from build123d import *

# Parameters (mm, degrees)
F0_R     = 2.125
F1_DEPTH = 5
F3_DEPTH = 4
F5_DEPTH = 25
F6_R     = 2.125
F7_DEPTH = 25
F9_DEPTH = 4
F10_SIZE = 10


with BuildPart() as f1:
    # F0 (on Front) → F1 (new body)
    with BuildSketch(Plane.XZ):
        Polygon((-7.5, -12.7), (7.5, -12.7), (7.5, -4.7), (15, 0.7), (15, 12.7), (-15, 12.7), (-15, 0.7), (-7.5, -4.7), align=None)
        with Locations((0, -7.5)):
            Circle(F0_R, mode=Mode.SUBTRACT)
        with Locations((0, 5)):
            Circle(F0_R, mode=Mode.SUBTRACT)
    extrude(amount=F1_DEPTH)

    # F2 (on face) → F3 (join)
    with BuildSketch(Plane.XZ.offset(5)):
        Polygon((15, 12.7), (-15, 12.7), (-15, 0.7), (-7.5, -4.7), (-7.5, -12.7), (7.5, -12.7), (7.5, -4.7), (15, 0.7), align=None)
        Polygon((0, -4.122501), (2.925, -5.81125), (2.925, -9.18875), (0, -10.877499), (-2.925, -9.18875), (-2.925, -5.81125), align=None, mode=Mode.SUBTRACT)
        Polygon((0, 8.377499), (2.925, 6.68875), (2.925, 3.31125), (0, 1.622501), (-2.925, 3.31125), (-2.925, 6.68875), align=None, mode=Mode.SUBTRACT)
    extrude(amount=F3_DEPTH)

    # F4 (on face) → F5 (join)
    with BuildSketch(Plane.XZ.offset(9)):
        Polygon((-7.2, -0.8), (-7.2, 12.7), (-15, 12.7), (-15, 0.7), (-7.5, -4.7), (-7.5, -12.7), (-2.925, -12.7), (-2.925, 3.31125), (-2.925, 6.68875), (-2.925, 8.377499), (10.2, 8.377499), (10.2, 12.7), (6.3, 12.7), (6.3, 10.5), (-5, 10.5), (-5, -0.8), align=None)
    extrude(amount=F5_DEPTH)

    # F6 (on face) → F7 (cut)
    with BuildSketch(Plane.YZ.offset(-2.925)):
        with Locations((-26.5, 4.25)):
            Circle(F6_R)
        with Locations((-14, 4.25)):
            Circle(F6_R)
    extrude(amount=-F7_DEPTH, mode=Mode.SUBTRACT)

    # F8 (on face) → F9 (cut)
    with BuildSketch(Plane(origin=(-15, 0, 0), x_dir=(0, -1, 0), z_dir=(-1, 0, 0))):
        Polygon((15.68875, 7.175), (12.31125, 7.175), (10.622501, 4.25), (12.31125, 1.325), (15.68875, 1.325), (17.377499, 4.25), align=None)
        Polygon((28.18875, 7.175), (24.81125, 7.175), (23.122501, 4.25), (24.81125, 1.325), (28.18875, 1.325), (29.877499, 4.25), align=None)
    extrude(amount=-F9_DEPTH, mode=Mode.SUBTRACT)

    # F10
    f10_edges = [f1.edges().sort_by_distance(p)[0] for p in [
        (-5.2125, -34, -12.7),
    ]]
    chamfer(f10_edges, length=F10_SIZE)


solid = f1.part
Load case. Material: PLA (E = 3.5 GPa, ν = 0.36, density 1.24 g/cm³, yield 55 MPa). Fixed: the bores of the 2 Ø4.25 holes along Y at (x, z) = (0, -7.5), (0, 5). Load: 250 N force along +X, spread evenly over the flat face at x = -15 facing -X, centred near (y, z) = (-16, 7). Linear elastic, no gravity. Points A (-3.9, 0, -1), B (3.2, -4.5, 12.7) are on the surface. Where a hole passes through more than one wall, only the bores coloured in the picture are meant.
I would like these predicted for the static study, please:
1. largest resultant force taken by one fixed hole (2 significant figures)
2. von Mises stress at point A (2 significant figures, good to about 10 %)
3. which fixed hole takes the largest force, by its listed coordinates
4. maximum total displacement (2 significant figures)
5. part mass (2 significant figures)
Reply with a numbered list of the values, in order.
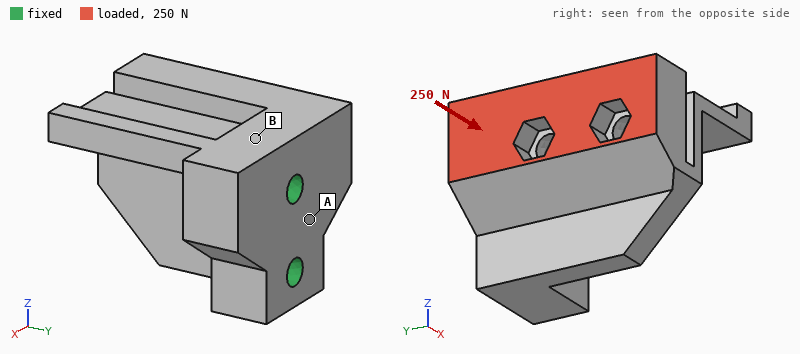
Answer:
1. 260 N
2. 8.0 MPa
3. (0, 5)
4. 0.55 mm
5. 13 g
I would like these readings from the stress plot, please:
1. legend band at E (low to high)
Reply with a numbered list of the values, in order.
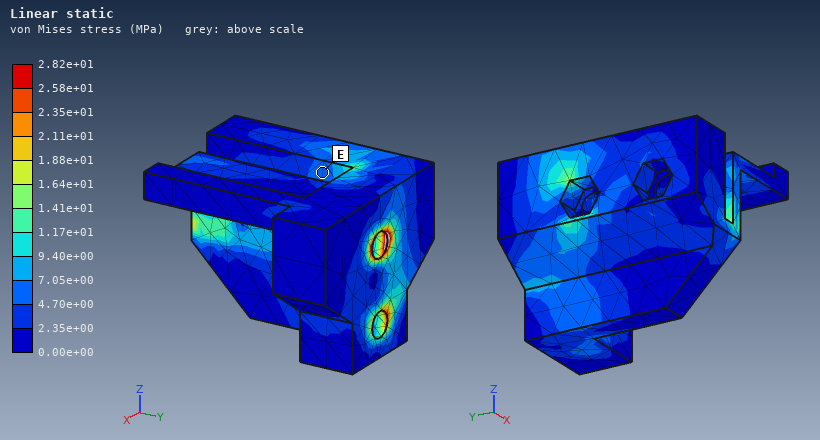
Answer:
1. 4.70e+00 to 7.05e+00 MPa
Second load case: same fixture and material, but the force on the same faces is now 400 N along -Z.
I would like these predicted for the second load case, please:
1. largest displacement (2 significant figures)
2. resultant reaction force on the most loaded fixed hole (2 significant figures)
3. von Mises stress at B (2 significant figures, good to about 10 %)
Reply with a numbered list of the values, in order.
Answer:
1. 0.32 mm
2. 570 N
3. 3.2 MPa
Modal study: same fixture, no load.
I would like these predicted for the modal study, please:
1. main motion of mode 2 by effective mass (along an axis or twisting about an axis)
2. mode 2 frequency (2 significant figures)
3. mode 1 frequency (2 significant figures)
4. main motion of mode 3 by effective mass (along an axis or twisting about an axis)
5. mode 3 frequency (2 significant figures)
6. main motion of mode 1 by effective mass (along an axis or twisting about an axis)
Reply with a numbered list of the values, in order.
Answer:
1. along Z
2. 2400 Hz
3. 1700 Hz
4. along Z
5. 3600 Hz
6. along X
